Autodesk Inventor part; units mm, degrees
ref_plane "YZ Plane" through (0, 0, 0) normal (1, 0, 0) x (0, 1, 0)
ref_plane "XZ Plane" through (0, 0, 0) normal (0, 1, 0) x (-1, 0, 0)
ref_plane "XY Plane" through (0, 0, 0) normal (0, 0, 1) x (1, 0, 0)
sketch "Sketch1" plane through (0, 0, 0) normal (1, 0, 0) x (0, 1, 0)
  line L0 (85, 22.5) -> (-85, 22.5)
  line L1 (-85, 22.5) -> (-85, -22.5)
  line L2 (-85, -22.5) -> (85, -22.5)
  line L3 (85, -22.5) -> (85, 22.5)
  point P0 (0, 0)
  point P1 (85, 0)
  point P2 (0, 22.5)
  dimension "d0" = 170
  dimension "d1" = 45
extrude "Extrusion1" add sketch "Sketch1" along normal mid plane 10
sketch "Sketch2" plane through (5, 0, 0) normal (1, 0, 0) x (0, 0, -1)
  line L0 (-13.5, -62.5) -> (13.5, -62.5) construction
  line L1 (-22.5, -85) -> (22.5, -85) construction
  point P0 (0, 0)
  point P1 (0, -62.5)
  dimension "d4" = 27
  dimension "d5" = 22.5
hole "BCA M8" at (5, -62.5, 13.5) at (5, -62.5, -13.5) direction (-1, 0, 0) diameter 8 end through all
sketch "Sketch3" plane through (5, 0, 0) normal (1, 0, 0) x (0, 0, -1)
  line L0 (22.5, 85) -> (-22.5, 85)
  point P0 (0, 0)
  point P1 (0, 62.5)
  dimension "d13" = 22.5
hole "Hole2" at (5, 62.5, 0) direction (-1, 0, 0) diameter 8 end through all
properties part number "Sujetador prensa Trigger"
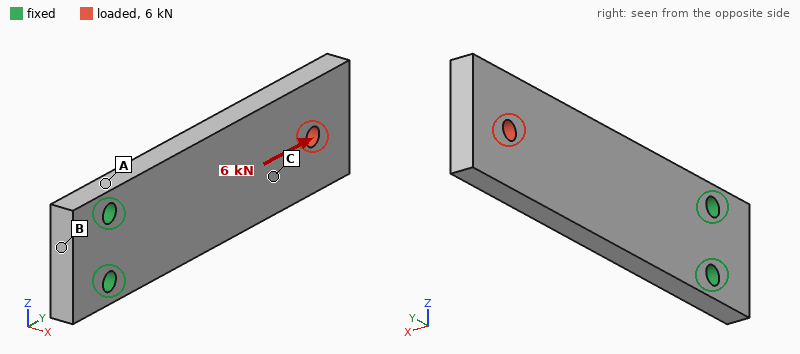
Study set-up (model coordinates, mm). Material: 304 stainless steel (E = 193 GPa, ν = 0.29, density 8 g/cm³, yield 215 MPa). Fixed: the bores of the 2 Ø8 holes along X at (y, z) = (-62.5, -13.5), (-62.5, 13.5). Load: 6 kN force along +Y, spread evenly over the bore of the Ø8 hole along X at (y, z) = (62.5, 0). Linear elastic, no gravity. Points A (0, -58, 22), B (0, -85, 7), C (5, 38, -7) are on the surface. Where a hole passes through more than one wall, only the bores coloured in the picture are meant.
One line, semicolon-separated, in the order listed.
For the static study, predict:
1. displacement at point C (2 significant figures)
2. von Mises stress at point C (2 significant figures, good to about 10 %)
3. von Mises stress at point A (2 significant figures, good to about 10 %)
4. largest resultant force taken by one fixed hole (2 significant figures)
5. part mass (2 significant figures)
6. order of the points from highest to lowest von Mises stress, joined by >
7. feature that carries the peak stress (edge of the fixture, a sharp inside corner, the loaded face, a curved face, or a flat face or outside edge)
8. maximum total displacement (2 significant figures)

7.0 µm; 15 MPa; 8.9 MPa; 3.0 kN; 600 g; C > A > B; the loaded face; 10 µm
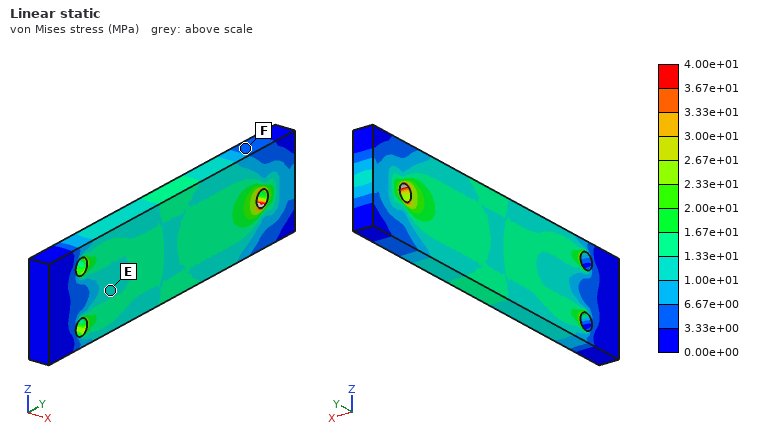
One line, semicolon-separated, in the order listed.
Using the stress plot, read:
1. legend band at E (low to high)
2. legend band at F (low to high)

1.00e+01 to 1.33e+01 MPa; 3.33e+00 to 6.67e+00 MPa
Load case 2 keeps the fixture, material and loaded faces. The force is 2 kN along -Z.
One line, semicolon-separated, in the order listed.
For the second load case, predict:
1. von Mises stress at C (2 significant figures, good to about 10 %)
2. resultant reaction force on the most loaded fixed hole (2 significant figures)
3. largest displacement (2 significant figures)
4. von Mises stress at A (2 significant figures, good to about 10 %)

11 MPa; 8.2 kN; 0.12 mm; 48 MPa
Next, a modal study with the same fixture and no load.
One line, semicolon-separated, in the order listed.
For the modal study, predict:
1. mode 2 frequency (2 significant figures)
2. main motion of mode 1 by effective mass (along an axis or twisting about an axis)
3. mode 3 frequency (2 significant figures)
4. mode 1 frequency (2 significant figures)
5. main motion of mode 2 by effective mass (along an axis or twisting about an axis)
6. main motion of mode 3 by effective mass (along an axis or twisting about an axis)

1600 Hz; along X; 2300 Hz; 380 Hz; along Z; twisting about Y
